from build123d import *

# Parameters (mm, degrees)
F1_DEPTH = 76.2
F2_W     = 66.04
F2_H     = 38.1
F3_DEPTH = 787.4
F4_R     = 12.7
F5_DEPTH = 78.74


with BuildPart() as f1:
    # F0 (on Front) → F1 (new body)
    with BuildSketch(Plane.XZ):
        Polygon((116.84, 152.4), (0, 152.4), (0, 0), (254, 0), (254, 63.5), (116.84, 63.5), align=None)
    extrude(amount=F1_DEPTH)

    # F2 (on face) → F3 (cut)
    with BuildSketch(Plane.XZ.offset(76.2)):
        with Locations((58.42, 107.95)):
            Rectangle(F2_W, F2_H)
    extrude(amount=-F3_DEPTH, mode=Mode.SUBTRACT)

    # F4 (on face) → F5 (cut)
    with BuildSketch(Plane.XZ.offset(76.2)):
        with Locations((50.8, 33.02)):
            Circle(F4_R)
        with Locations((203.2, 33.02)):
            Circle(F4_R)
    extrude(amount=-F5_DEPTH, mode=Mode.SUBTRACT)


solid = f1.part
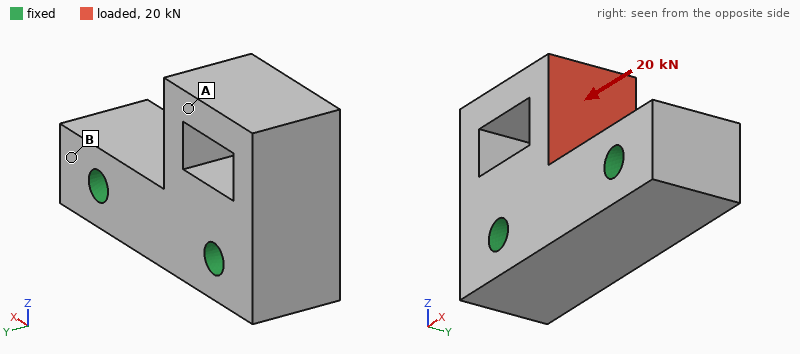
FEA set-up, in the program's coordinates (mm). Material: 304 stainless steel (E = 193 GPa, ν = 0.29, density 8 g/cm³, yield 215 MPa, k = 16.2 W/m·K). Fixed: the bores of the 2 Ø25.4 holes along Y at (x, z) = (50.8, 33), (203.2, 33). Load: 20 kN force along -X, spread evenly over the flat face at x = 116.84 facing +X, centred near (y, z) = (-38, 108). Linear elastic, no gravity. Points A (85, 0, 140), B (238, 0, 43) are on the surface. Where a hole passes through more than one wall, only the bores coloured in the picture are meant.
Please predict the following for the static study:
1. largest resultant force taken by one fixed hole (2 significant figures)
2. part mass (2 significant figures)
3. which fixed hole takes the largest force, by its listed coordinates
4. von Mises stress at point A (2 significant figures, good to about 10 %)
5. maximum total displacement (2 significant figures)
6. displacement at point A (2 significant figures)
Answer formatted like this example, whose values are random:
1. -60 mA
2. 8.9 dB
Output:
1. 17 kN
2. 14 kg
3. (50.8, 33)
4. 5.2 MPa
5. 19 µm
6. 16 µm
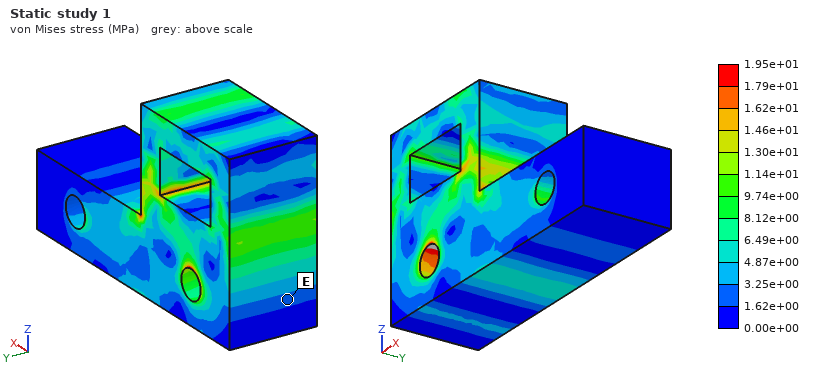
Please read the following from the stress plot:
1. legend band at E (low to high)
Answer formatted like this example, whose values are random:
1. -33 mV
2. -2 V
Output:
1. 1.62e+00 to 3.25e+00 MPa
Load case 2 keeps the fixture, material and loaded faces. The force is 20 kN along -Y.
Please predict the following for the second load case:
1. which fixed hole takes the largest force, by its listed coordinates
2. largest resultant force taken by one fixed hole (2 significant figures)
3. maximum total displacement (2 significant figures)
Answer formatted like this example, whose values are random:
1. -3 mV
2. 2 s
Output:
1. (50.8, 33)
2. 15 kN
3. 31 µm
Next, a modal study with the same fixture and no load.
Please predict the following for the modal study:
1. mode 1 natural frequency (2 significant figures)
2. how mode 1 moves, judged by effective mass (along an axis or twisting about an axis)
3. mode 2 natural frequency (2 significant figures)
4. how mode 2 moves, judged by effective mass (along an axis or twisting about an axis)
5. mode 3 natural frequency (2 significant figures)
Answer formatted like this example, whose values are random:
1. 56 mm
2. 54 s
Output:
1. 2700 Hz
2. along X
3. 2900 Hz
4. along Y
5. 4500 Hz
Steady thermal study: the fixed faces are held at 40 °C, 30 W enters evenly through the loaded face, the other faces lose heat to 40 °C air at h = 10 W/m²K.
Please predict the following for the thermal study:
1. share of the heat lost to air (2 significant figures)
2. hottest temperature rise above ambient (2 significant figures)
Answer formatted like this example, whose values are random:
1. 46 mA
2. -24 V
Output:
1. 24 %
2. 30 K
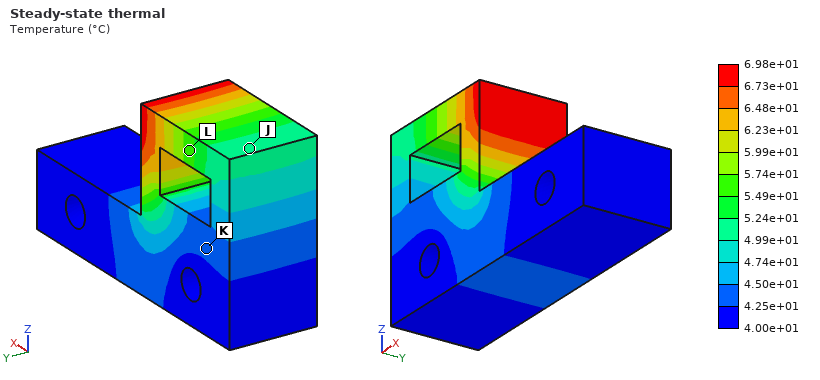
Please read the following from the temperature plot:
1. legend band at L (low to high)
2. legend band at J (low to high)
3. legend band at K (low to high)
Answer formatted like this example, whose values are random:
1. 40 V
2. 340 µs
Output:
1. 5.49e+01 to 5.74e+01 °C
2. 4.99e+01 to 5.24e+01 °C
3. 4.25e+01 to 4.50e+01 °C
